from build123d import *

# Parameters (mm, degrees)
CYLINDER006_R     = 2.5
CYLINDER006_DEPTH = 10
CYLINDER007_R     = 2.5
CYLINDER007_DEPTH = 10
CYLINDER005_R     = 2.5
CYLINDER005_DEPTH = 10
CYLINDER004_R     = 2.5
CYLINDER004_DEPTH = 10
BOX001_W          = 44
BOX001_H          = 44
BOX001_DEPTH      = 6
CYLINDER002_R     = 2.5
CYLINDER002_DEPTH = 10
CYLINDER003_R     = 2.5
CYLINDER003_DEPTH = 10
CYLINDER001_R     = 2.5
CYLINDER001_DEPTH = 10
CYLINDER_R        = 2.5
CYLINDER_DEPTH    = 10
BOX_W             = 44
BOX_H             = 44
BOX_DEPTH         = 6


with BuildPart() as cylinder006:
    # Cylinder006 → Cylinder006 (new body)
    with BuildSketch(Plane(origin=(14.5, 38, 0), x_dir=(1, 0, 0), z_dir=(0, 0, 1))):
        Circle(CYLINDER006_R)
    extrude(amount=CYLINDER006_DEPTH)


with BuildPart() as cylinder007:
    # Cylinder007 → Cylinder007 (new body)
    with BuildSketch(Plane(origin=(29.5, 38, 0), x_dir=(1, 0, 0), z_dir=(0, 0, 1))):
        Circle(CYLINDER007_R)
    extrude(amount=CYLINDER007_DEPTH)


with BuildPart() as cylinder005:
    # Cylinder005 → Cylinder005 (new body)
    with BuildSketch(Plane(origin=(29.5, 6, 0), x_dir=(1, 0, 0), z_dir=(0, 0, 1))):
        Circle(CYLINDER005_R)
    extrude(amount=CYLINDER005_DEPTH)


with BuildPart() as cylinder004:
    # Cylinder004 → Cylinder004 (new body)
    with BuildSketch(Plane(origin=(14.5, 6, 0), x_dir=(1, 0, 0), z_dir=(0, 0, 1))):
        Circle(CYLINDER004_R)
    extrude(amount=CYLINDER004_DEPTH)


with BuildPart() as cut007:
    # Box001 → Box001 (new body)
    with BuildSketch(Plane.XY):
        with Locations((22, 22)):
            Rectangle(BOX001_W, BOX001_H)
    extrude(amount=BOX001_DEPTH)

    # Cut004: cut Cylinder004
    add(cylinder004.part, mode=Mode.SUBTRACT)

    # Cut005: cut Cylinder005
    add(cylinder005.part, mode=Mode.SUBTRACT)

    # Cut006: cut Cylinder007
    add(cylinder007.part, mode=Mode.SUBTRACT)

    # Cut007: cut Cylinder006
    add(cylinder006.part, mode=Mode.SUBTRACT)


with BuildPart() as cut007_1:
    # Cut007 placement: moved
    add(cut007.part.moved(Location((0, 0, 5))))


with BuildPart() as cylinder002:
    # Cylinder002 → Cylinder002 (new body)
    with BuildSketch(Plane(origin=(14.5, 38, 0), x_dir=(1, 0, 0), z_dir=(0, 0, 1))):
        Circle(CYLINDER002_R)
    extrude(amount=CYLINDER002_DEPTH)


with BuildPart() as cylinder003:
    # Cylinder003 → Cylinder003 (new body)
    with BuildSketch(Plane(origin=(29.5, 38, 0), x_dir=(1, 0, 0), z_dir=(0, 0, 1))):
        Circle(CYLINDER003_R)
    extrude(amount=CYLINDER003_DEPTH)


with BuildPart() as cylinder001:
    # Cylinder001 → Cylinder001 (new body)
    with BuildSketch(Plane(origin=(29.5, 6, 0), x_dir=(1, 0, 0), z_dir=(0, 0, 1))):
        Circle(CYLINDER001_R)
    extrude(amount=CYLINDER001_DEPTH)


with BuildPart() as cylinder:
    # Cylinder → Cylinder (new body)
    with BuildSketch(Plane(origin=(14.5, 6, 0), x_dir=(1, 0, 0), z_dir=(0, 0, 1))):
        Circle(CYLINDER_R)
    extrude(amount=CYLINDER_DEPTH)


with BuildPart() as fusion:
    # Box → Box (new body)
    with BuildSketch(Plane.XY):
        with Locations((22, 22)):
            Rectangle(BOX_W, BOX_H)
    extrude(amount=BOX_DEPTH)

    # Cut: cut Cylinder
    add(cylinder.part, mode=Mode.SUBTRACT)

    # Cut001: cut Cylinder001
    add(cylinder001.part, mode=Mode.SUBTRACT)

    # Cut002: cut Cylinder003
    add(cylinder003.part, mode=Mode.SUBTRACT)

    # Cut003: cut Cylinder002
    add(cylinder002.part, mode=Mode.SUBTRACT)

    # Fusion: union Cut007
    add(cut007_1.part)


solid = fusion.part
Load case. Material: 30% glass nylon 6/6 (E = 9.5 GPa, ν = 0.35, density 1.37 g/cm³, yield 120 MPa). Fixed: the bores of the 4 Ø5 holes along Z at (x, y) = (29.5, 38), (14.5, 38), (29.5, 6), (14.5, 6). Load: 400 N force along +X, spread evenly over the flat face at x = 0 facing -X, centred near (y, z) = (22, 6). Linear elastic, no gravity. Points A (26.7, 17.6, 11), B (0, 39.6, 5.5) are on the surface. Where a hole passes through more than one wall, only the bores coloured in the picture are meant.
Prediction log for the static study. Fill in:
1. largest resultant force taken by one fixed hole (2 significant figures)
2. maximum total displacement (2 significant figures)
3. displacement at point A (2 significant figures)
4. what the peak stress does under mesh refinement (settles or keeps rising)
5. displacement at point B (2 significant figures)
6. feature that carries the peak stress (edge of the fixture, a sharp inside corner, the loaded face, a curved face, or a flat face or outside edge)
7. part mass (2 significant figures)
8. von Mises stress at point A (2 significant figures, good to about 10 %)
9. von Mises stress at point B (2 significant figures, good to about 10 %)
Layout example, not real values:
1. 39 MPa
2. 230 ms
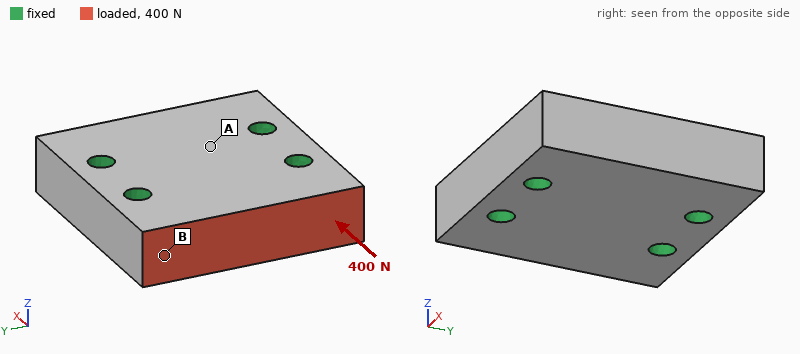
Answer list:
1. 160 N
2. 1.9 µm
3. 0.53 µm
4. keeps rising
5. 1.3 µm
6. edge of the fixture
7. 28 g
8. 0.24 MPa
9. 0.87 MPa
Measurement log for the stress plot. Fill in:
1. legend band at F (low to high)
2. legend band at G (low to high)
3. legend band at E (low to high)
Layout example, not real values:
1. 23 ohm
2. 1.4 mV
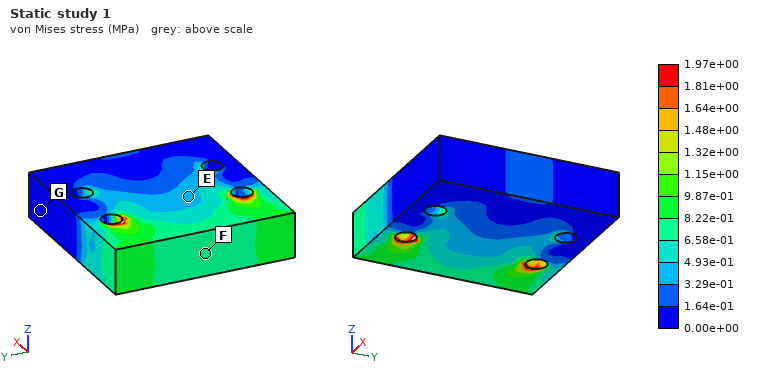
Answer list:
1. 6.58e-01 to 8.22e-01 MPa
2. 0.00e+00 to 1.64e-01 MPa
3. 3.29e-01 to 4.93e-01 MPa
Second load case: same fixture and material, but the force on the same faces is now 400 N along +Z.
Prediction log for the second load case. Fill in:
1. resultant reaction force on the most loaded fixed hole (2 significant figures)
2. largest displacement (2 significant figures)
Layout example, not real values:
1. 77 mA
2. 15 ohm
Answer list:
1. 240 N
2. 19 µm
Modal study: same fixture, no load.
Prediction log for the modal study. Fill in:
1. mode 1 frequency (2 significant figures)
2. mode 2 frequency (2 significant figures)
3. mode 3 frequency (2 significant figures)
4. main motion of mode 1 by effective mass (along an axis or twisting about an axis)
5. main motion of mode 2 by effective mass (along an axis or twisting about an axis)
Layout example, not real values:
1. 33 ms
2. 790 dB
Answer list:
1. 13 kHz
2. 14 kHz
3. 20 kHz
4. twisting about Y
5. along Z
